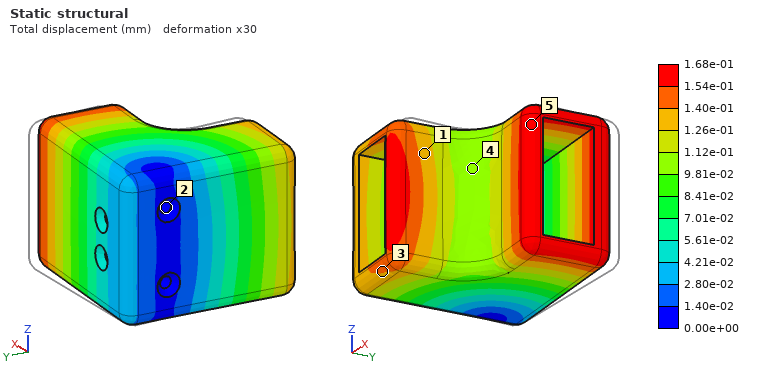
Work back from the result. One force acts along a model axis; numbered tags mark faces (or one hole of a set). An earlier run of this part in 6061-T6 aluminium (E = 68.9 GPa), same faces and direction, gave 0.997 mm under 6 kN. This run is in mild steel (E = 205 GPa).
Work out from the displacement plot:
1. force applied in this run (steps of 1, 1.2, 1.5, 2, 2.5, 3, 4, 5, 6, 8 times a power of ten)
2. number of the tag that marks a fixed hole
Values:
3 kN
2
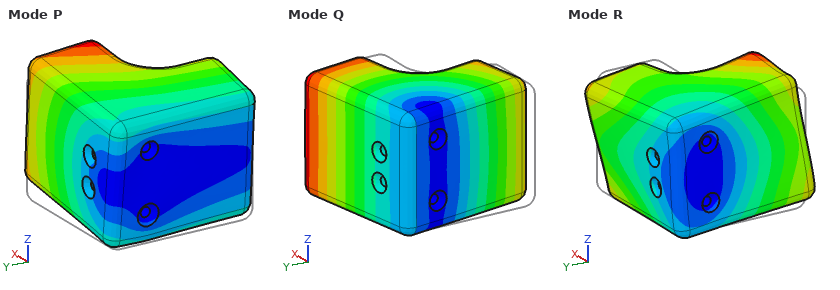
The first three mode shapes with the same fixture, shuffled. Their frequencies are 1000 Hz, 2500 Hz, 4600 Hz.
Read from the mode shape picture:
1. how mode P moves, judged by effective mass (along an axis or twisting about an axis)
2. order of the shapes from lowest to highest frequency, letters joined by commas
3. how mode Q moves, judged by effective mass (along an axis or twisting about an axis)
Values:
along Z
Q, P, R
along Y
